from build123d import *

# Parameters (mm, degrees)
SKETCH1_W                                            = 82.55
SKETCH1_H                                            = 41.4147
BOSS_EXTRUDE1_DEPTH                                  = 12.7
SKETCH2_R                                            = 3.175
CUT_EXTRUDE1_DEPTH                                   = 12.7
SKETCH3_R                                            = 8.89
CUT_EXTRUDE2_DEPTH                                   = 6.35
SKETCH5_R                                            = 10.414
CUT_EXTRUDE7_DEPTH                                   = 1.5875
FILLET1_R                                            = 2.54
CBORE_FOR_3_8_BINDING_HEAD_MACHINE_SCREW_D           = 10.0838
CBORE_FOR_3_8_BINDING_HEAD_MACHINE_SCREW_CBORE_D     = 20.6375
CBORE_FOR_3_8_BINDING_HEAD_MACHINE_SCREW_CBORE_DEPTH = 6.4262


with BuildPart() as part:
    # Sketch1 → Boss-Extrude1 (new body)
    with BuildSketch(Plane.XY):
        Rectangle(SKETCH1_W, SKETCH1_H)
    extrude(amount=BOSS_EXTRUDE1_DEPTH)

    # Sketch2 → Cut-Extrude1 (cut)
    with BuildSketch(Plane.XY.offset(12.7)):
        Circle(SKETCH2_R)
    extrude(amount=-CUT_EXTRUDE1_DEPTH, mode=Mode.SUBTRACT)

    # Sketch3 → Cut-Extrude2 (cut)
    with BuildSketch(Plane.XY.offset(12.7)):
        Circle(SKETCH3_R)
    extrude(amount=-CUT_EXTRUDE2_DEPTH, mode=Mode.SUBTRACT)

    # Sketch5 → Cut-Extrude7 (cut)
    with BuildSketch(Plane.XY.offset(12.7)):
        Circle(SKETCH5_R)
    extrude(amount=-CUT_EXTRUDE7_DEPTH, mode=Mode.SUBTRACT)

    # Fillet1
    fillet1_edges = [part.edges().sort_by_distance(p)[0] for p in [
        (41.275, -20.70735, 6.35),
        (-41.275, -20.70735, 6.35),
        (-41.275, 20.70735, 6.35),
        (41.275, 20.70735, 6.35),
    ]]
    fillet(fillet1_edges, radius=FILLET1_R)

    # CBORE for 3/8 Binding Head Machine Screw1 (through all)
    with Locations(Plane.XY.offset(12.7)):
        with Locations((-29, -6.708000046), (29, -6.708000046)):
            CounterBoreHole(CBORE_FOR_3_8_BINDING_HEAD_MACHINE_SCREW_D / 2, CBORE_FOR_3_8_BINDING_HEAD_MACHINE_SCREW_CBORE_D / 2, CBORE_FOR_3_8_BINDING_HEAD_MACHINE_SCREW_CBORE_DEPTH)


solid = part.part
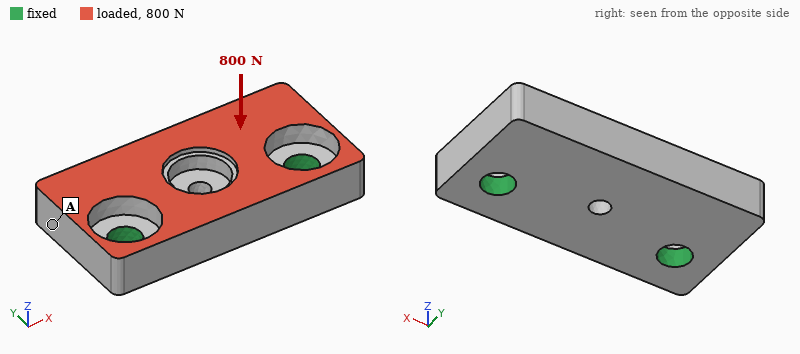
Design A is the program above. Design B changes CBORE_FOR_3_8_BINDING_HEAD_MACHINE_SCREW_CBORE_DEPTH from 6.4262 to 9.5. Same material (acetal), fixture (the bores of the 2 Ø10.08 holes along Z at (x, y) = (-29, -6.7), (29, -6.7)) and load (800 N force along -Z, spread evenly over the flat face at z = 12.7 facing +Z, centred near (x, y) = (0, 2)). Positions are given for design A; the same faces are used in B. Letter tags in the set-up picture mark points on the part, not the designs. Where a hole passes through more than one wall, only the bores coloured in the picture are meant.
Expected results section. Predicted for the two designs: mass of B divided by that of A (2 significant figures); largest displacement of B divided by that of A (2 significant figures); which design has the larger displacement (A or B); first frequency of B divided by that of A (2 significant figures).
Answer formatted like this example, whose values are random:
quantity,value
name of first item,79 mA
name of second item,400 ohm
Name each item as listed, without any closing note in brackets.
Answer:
quantity,value
mass of B divided by that of A,0.96
largest displacement of B divided by that of A,2.3
which design has the larger displacement,B
first frequency of B divided by that of A,0.61
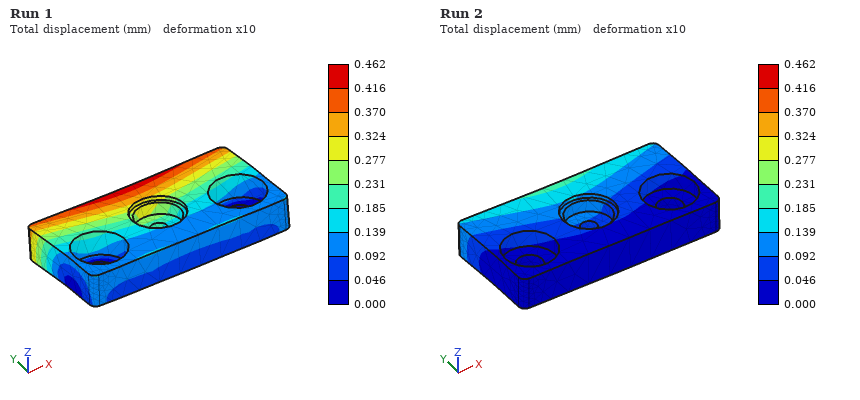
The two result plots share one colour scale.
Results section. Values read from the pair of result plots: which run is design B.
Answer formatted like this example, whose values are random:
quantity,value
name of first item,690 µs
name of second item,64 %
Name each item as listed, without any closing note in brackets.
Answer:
quantity,value
which run is design B,Run 1
